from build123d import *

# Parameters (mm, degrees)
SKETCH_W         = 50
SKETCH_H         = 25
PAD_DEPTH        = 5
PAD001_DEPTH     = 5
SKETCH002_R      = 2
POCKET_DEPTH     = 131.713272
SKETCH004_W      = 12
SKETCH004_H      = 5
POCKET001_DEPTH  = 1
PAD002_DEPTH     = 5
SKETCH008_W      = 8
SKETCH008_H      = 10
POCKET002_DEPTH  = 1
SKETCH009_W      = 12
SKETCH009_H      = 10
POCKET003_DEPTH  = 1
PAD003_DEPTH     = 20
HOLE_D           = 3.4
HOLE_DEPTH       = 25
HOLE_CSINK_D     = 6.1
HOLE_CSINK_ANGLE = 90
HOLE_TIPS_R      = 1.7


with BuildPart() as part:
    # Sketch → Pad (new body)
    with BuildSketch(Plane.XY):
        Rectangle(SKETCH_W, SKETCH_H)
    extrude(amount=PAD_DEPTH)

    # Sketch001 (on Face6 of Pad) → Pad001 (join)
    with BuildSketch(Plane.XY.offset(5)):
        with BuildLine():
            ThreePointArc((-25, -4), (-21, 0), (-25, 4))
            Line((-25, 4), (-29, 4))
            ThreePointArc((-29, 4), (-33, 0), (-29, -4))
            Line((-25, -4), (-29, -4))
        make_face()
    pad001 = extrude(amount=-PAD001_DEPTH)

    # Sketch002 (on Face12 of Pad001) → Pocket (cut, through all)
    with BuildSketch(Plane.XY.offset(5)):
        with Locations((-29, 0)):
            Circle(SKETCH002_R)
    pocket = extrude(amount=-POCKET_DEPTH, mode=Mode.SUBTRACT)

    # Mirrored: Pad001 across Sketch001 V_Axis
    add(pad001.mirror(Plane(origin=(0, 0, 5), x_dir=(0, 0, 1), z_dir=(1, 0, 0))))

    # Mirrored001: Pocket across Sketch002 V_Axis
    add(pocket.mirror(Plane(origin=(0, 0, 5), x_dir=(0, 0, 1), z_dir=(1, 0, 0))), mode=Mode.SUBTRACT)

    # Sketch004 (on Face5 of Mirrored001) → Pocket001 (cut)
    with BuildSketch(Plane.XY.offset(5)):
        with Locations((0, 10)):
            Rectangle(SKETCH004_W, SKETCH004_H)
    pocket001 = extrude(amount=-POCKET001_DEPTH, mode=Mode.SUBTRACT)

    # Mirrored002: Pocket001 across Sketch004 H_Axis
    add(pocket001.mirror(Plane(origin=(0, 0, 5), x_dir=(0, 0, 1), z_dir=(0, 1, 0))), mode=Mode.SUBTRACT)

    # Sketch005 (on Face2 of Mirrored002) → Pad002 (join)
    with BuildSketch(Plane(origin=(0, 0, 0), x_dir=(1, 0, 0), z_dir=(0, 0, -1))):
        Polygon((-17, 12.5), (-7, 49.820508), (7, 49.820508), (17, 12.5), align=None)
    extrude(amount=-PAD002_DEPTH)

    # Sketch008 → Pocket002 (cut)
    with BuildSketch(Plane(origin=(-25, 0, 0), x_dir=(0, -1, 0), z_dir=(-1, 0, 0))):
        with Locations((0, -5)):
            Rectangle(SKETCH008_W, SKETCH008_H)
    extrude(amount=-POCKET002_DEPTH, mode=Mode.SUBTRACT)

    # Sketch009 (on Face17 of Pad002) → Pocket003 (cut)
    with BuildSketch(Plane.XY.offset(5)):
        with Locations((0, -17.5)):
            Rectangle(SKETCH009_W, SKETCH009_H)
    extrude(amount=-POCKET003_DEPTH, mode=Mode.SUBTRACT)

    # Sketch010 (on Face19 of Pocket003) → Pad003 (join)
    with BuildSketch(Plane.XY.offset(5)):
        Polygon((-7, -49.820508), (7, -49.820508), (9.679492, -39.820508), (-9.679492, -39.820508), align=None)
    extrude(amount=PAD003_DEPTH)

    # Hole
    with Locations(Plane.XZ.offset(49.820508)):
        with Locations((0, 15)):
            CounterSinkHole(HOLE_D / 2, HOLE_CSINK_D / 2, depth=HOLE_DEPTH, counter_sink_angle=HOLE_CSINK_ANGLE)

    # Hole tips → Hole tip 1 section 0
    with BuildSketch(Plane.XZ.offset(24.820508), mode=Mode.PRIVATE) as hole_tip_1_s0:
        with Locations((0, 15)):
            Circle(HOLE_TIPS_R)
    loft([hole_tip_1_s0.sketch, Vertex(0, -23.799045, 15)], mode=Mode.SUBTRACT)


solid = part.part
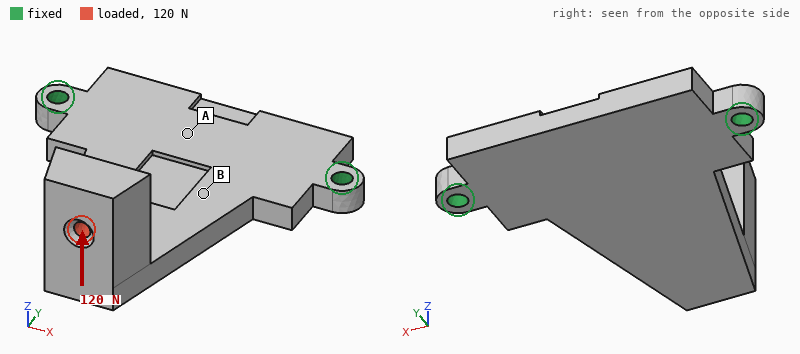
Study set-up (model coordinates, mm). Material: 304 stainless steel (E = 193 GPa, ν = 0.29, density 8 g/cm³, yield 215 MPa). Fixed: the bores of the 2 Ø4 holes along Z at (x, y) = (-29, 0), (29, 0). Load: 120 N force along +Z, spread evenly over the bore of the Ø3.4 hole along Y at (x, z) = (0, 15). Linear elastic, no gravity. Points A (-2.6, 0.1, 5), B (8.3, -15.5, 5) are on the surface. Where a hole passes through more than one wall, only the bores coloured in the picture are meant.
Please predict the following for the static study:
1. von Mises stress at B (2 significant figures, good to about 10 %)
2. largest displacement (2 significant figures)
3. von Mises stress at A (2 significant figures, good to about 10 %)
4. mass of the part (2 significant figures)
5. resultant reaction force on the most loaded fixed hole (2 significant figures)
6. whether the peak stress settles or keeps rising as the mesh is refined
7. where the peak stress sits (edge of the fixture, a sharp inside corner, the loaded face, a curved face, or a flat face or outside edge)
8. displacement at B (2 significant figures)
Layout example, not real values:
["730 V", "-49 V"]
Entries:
["34 MPa", "0.13 mm", "11 MPa", "110 g", "60 N", "keeps rising", "edge of the fixture", "0.026 mm"]
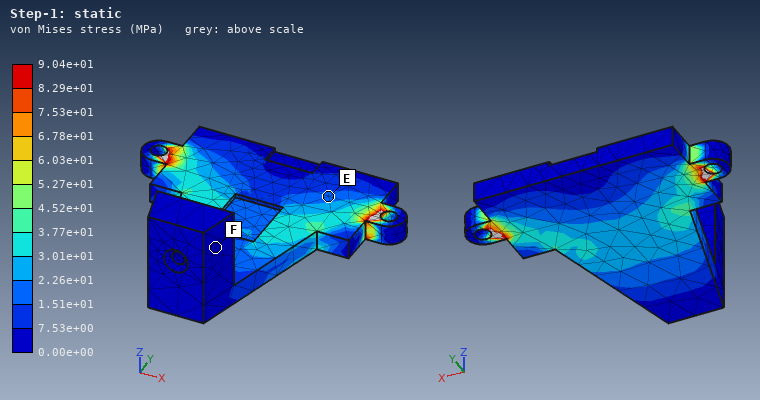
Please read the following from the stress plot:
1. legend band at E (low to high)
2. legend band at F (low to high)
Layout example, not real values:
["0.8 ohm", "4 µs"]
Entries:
["1.51e+01 to 2.26e+01 MPa", "0.00e+00 to 7.53e+00 MPa"]
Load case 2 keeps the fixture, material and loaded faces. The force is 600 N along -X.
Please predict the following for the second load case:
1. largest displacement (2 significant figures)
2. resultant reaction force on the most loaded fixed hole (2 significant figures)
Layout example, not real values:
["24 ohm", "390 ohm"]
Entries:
["92 µm", "600 N"]
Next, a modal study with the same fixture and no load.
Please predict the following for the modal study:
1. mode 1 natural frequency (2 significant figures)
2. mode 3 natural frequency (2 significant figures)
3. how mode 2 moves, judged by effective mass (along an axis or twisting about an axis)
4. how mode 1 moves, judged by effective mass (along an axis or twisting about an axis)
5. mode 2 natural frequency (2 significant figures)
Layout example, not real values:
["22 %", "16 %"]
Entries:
["810 Hz", "3600 Hz", "along X", "along Z", "2800 Hz"]
